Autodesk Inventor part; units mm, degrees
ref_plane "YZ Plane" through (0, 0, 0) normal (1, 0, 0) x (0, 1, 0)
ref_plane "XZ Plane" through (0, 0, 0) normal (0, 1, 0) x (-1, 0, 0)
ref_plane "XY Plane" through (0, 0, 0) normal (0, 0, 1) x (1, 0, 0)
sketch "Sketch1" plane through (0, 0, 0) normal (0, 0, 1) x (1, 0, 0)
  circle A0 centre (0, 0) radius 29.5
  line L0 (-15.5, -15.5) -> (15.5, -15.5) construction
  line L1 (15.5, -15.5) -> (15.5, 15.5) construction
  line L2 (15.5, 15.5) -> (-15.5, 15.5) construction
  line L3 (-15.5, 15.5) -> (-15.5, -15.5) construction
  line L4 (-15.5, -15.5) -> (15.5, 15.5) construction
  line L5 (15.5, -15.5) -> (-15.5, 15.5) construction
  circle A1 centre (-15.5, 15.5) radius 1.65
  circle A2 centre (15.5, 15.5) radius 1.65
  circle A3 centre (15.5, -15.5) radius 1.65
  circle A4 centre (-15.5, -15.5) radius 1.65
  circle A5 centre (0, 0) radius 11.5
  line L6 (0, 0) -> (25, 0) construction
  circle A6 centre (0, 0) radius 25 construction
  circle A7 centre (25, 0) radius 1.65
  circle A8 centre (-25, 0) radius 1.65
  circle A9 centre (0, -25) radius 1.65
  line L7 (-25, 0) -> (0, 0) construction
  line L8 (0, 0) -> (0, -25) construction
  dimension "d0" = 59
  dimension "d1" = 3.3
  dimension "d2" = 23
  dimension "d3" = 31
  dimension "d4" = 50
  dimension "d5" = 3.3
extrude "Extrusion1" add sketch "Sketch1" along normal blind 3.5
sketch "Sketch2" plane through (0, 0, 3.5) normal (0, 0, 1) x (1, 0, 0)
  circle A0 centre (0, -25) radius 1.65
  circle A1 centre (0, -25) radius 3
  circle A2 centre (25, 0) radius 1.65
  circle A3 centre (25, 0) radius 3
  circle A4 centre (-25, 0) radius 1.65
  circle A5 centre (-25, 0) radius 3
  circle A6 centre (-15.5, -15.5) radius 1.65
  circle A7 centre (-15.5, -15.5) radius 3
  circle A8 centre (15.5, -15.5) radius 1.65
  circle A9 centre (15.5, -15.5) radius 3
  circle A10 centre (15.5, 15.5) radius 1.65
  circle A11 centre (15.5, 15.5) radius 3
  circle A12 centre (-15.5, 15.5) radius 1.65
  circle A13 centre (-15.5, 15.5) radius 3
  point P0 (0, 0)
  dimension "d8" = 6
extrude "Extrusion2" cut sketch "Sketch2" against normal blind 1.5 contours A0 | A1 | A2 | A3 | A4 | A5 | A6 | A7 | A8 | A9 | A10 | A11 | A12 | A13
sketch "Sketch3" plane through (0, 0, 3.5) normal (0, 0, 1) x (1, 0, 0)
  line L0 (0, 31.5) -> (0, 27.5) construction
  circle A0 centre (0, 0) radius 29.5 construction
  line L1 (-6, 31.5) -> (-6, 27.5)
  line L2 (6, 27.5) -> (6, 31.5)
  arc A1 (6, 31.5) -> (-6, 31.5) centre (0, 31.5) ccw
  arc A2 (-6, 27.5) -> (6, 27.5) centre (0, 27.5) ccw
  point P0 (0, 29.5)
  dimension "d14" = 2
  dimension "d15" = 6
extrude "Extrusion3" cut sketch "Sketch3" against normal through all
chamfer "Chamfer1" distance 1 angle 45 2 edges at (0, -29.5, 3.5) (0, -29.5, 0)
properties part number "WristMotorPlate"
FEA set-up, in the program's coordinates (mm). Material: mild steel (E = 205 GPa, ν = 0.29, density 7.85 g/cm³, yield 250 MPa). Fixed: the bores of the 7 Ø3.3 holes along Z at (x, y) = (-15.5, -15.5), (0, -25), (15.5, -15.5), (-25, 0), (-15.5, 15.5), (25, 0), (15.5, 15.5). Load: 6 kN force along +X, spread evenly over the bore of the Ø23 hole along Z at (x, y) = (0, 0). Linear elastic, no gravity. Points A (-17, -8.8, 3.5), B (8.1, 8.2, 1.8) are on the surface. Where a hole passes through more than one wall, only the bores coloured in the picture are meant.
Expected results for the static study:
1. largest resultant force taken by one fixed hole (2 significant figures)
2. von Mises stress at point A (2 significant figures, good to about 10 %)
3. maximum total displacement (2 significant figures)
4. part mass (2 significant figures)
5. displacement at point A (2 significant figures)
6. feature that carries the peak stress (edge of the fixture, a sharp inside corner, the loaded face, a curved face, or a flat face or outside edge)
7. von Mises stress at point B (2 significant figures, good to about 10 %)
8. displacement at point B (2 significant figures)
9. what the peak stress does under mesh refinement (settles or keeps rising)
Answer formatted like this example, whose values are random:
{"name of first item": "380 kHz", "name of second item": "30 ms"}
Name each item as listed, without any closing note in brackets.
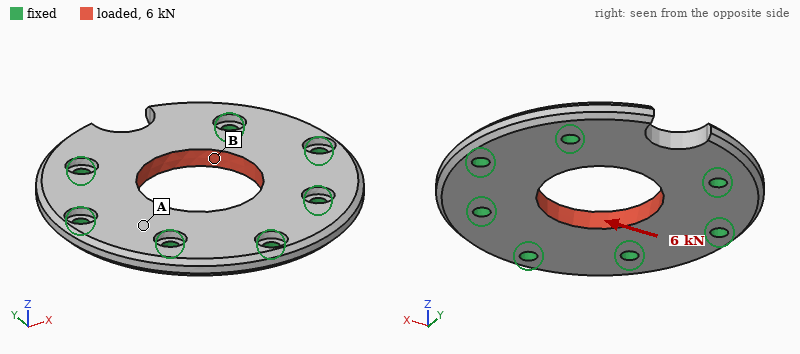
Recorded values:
{"largest resultant force taken by one fixed hole": "1.0 kN", "von Mises stress at point A": "13 MPa", "maximum total displacement": "3.2 µm", "part mass": "57 g", "displacement at point A": "1.6 µm", "feature that carries the peak stress": "edge of the fixture", "von Mises stress at point B": "34 MPa", "displacement at point B": "2.6 µm", "what the peak stress does under mesh refinement": "keeps rising"}
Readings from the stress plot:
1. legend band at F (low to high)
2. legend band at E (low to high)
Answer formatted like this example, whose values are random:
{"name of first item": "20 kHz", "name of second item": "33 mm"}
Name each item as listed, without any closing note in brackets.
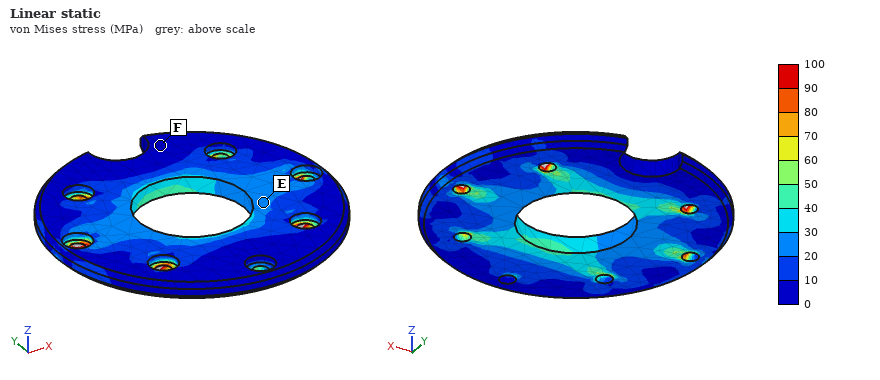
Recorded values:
{"legend band at F": "0 to 10 MPa", "legend band at E": "20 to 30 MPa"}
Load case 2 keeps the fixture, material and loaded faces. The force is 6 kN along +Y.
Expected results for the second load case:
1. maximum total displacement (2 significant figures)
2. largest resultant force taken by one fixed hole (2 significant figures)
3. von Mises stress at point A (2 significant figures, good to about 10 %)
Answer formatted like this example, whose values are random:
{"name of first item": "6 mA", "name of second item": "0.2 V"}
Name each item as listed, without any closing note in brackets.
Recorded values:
{"maximum total displacement": "5.7 µm", "largest resultant force taken by one fixed hole": "1.3 kN", "von Mises stress at point A": "13 MPa"}
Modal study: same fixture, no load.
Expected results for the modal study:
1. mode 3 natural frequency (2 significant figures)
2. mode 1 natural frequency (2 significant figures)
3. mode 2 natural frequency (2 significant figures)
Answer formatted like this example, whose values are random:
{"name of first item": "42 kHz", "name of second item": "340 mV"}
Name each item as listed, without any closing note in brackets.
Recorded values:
{"mode 3 natural frequency": "21 kHz", "mode 1 natural frequency": "13 kHz", "mode 2 natural frequency": "17 kHz"}
